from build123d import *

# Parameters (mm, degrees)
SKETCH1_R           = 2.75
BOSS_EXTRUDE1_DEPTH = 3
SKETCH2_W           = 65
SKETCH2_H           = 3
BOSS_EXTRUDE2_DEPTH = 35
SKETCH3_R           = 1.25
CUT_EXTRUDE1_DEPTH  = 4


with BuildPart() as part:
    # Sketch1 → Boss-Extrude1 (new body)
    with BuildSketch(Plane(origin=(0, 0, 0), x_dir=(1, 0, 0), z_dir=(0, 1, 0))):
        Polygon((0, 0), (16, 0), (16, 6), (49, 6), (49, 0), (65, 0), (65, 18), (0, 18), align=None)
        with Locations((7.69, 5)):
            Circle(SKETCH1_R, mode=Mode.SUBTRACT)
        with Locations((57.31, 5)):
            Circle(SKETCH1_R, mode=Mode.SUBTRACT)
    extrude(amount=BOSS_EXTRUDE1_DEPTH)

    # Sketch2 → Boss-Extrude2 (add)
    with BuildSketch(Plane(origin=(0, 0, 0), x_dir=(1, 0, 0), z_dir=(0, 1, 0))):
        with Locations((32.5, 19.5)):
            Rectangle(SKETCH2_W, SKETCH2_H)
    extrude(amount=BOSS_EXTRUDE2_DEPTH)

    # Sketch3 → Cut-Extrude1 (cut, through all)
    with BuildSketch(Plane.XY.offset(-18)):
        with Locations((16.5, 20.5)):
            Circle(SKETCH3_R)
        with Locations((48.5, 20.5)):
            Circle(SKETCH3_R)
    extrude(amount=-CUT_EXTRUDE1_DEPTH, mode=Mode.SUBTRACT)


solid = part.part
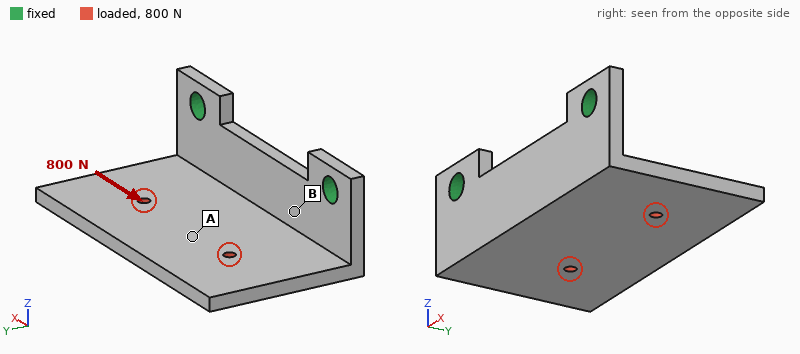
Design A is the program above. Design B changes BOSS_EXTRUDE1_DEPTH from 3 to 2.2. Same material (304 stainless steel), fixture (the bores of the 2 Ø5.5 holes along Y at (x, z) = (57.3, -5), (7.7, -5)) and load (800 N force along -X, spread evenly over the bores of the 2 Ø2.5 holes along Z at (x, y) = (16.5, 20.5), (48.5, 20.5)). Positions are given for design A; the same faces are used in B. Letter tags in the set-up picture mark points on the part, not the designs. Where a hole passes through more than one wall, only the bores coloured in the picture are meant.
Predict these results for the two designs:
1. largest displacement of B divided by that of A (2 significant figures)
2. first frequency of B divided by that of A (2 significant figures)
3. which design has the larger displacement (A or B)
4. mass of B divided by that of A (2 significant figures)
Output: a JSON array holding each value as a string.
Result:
["1.8", "0.68", "B", "0.92"]
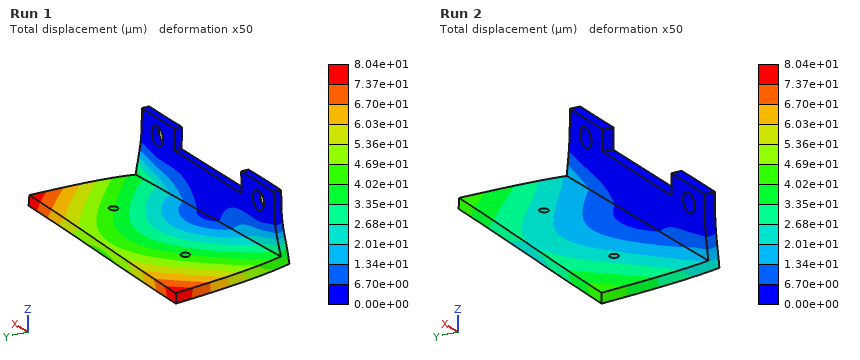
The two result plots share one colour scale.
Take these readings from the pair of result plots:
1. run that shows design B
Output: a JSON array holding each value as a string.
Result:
["Run 1"]
